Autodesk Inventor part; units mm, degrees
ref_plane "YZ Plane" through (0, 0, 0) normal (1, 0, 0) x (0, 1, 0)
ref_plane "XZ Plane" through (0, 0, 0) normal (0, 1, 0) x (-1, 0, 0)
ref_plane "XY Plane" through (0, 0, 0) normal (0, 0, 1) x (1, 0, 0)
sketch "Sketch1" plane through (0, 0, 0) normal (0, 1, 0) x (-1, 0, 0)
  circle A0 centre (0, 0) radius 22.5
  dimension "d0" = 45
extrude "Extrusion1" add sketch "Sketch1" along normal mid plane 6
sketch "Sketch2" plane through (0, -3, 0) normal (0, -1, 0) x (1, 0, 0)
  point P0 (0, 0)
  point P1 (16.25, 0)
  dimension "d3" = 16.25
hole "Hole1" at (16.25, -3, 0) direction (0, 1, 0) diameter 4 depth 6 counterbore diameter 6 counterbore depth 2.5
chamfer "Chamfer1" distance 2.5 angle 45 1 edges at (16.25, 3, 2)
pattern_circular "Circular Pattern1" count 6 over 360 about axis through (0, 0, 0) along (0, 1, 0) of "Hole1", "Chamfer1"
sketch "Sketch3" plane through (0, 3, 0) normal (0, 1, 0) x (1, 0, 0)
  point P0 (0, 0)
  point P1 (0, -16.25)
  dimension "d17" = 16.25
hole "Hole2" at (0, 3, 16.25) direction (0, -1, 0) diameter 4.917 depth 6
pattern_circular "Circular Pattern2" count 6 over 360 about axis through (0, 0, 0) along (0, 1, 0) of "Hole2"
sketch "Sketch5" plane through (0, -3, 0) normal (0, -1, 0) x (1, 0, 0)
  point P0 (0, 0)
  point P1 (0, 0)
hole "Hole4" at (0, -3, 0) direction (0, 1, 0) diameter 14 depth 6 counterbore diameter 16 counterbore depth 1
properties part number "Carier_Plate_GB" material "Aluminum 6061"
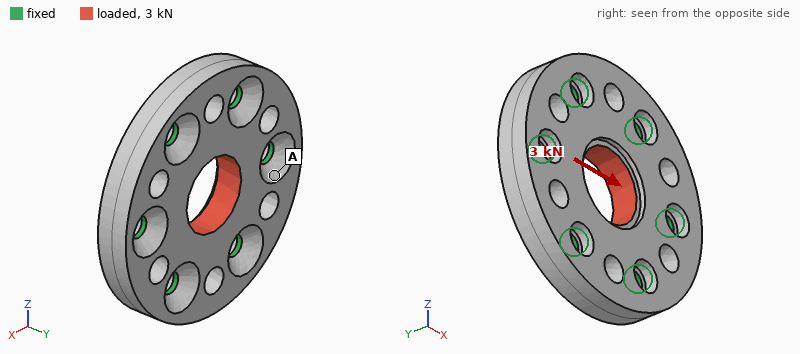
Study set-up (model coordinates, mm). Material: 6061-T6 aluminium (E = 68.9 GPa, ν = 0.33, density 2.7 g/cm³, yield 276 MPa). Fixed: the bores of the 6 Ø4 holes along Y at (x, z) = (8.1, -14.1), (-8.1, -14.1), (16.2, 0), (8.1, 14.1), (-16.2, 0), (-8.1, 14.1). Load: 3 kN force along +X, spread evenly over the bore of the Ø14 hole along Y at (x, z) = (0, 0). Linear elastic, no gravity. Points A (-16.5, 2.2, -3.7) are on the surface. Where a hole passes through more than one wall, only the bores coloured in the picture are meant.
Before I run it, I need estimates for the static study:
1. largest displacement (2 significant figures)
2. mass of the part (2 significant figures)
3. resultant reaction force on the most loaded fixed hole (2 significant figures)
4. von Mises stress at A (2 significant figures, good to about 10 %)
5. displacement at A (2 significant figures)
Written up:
3.2 µm
19 g
690 N
12 MPa
1.3 µm
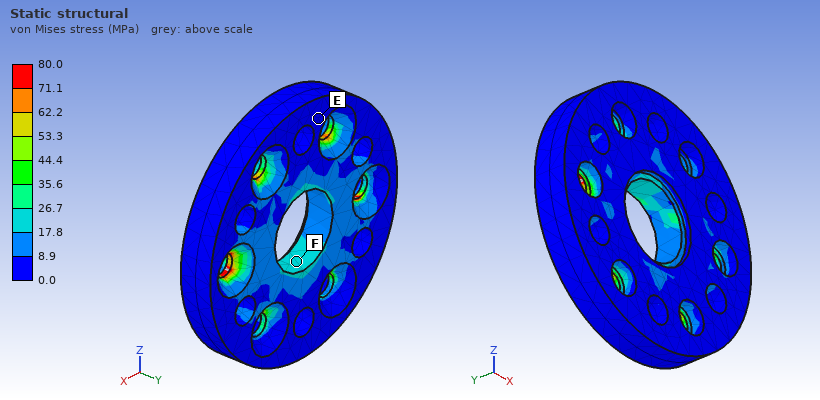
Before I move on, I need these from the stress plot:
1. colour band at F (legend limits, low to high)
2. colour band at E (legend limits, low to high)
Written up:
17.8 to 26.7 MPa
0.0 to 8.9 MPa
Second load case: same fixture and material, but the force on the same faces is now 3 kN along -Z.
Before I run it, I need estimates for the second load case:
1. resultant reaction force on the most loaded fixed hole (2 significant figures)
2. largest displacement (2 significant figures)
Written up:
620 N
3.3 µm
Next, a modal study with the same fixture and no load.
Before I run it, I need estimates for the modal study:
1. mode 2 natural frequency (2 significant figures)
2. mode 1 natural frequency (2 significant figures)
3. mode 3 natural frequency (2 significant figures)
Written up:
29 kHz
26 kHz
30 kHz
